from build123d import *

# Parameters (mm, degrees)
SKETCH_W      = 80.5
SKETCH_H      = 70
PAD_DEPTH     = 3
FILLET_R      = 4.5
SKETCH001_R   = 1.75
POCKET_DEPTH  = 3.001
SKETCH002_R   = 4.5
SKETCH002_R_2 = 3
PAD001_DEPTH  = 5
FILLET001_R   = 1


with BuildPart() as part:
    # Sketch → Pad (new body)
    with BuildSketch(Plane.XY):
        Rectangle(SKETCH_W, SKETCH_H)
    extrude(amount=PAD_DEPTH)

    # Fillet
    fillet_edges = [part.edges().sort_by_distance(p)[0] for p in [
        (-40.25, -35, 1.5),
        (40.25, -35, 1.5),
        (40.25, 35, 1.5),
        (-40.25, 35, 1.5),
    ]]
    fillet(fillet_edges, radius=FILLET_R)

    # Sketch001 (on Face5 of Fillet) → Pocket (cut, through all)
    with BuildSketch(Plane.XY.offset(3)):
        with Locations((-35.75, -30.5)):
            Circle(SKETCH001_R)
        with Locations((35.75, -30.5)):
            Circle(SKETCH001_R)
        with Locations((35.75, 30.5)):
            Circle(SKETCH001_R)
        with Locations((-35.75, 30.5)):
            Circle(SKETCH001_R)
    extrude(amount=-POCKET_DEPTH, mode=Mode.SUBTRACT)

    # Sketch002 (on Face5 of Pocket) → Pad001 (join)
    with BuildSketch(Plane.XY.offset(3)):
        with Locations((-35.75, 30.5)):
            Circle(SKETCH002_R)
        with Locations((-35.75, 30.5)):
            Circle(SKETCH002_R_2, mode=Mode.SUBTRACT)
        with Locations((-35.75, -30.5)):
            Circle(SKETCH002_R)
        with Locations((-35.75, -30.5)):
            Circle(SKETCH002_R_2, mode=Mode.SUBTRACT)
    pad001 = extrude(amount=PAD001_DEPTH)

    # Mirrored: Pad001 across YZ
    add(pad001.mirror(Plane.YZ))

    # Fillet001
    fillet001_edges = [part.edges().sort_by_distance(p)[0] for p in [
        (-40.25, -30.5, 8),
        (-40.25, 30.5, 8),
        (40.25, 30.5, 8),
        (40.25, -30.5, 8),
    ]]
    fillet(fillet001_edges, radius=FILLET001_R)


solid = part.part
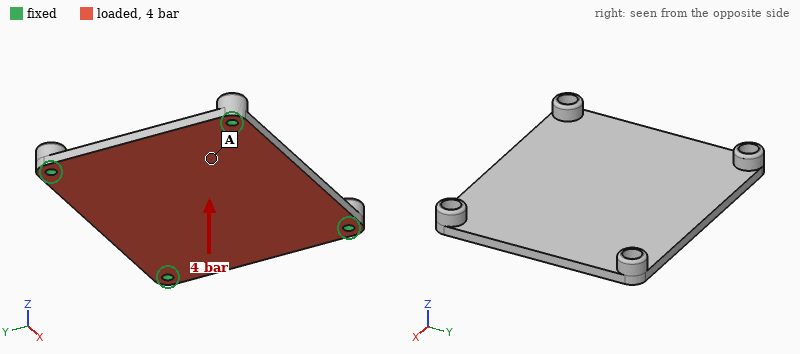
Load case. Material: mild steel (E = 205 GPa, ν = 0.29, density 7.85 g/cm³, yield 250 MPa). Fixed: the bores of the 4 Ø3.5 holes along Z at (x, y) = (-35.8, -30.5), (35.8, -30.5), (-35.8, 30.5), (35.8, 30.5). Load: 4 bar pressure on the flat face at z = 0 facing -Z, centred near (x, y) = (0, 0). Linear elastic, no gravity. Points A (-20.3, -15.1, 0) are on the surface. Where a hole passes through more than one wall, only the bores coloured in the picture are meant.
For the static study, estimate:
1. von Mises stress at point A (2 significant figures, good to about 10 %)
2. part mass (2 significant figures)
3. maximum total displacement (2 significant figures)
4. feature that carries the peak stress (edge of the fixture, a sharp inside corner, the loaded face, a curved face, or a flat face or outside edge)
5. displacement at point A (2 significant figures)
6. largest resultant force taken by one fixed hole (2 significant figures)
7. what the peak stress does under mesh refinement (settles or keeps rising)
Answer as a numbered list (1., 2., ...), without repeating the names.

1. 34 MPa
2. 140 g
3. 0.12 mm
4. edge of the fixture
5. 0.073 mm
6. 560 N
7. keeps rising
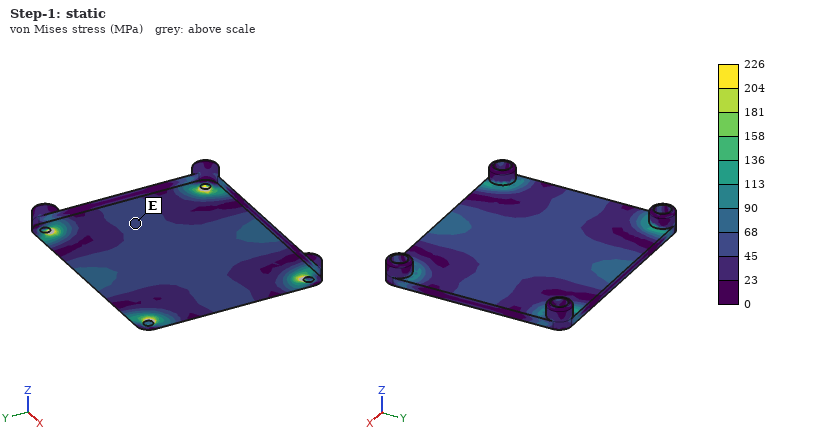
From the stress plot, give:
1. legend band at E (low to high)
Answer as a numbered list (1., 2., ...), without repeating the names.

1. 45 to 68 MPa
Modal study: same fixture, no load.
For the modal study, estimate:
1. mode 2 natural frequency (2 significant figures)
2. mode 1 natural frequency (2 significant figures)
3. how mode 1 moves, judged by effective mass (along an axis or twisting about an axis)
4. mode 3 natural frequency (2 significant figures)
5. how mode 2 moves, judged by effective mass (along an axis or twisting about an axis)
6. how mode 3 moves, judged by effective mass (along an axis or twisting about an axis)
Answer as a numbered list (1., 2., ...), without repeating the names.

1. 3700 Hz
2. 2300 Hz
3. along Z
4. 4500 Hz
5. twisting about X
6. twisting about Y
